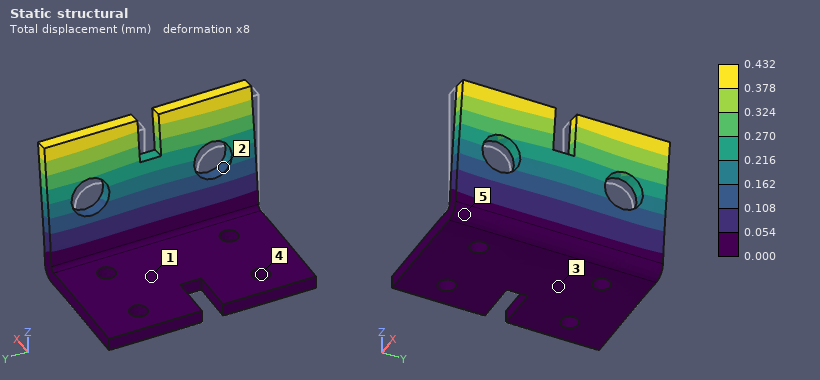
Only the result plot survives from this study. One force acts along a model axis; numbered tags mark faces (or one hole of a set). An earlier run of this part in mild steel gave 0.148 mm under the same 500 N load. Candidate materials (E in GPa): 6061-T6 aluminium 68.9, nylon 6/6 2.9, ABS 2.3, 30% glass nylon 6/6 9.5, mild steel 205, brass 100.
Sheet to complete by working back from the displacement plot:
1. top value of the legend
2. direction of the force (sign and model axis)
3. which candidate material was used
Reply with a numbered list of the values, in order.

1. 0.432 mm
2. +X
3. 6061-T6 aluminium
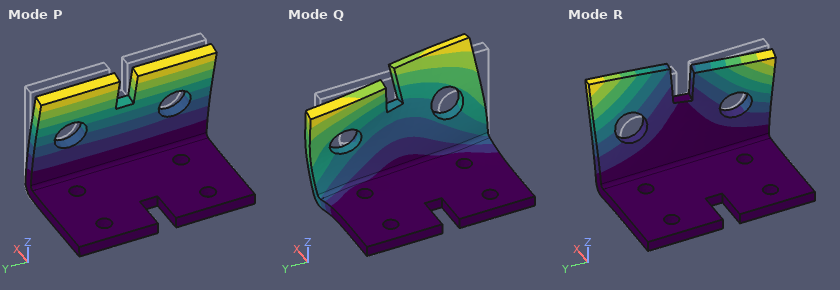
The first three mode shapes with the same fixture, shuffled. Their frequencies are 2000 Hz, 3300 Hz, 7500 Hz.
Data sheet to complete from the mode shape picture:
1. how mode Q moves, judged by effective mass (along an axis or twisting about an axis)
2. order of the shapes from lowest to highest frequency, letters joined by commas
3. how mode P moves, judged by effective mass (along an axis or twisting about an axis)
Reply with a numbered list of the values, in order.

1. along Y
2. P, R, Q
3. along X
